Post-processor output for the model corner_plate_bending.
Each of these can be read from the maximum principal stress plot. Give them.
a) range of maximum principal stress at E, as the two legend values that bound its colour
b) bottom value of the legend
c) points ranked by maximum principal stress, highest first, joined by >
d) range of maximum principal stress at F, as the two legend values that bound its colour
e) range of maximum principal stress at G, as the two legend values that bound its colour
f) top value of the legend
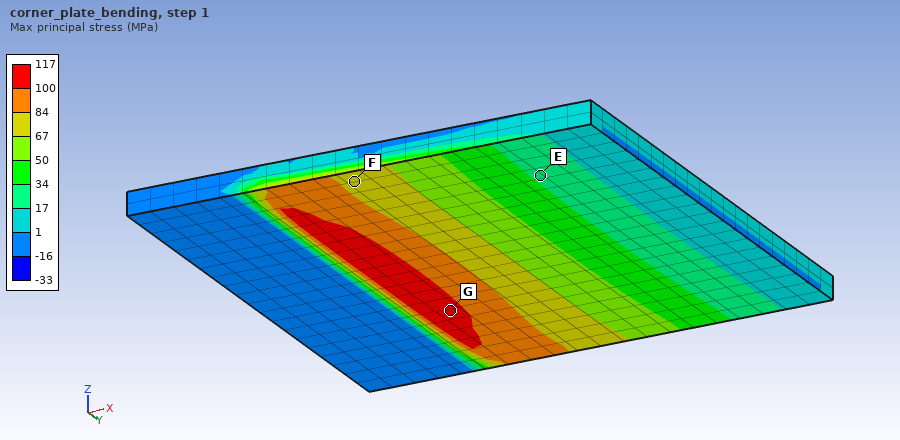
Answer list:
17 to 34 MPa
-33 MPa
G > F > E
67 to 84 MPa
100 to 117 MPa
117 MPa
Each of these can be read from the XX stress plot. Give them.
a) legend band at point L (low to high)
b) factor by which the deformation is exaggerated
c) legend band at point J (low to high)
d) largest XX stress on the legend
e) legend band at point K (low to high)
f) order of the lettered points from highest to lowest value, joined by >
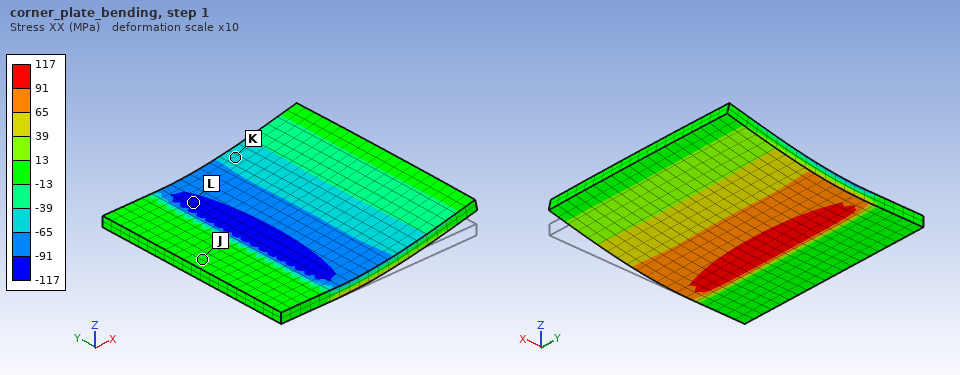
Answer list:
-117 to -91 MPa
10
-13 to 13 MPa
117 MPa
-65 to -39 MPa
J > K > L
